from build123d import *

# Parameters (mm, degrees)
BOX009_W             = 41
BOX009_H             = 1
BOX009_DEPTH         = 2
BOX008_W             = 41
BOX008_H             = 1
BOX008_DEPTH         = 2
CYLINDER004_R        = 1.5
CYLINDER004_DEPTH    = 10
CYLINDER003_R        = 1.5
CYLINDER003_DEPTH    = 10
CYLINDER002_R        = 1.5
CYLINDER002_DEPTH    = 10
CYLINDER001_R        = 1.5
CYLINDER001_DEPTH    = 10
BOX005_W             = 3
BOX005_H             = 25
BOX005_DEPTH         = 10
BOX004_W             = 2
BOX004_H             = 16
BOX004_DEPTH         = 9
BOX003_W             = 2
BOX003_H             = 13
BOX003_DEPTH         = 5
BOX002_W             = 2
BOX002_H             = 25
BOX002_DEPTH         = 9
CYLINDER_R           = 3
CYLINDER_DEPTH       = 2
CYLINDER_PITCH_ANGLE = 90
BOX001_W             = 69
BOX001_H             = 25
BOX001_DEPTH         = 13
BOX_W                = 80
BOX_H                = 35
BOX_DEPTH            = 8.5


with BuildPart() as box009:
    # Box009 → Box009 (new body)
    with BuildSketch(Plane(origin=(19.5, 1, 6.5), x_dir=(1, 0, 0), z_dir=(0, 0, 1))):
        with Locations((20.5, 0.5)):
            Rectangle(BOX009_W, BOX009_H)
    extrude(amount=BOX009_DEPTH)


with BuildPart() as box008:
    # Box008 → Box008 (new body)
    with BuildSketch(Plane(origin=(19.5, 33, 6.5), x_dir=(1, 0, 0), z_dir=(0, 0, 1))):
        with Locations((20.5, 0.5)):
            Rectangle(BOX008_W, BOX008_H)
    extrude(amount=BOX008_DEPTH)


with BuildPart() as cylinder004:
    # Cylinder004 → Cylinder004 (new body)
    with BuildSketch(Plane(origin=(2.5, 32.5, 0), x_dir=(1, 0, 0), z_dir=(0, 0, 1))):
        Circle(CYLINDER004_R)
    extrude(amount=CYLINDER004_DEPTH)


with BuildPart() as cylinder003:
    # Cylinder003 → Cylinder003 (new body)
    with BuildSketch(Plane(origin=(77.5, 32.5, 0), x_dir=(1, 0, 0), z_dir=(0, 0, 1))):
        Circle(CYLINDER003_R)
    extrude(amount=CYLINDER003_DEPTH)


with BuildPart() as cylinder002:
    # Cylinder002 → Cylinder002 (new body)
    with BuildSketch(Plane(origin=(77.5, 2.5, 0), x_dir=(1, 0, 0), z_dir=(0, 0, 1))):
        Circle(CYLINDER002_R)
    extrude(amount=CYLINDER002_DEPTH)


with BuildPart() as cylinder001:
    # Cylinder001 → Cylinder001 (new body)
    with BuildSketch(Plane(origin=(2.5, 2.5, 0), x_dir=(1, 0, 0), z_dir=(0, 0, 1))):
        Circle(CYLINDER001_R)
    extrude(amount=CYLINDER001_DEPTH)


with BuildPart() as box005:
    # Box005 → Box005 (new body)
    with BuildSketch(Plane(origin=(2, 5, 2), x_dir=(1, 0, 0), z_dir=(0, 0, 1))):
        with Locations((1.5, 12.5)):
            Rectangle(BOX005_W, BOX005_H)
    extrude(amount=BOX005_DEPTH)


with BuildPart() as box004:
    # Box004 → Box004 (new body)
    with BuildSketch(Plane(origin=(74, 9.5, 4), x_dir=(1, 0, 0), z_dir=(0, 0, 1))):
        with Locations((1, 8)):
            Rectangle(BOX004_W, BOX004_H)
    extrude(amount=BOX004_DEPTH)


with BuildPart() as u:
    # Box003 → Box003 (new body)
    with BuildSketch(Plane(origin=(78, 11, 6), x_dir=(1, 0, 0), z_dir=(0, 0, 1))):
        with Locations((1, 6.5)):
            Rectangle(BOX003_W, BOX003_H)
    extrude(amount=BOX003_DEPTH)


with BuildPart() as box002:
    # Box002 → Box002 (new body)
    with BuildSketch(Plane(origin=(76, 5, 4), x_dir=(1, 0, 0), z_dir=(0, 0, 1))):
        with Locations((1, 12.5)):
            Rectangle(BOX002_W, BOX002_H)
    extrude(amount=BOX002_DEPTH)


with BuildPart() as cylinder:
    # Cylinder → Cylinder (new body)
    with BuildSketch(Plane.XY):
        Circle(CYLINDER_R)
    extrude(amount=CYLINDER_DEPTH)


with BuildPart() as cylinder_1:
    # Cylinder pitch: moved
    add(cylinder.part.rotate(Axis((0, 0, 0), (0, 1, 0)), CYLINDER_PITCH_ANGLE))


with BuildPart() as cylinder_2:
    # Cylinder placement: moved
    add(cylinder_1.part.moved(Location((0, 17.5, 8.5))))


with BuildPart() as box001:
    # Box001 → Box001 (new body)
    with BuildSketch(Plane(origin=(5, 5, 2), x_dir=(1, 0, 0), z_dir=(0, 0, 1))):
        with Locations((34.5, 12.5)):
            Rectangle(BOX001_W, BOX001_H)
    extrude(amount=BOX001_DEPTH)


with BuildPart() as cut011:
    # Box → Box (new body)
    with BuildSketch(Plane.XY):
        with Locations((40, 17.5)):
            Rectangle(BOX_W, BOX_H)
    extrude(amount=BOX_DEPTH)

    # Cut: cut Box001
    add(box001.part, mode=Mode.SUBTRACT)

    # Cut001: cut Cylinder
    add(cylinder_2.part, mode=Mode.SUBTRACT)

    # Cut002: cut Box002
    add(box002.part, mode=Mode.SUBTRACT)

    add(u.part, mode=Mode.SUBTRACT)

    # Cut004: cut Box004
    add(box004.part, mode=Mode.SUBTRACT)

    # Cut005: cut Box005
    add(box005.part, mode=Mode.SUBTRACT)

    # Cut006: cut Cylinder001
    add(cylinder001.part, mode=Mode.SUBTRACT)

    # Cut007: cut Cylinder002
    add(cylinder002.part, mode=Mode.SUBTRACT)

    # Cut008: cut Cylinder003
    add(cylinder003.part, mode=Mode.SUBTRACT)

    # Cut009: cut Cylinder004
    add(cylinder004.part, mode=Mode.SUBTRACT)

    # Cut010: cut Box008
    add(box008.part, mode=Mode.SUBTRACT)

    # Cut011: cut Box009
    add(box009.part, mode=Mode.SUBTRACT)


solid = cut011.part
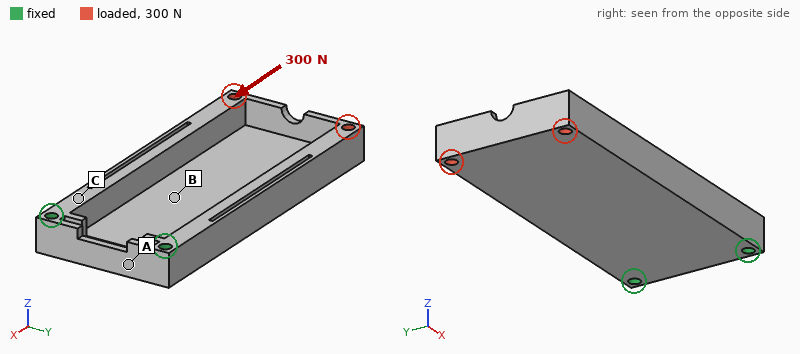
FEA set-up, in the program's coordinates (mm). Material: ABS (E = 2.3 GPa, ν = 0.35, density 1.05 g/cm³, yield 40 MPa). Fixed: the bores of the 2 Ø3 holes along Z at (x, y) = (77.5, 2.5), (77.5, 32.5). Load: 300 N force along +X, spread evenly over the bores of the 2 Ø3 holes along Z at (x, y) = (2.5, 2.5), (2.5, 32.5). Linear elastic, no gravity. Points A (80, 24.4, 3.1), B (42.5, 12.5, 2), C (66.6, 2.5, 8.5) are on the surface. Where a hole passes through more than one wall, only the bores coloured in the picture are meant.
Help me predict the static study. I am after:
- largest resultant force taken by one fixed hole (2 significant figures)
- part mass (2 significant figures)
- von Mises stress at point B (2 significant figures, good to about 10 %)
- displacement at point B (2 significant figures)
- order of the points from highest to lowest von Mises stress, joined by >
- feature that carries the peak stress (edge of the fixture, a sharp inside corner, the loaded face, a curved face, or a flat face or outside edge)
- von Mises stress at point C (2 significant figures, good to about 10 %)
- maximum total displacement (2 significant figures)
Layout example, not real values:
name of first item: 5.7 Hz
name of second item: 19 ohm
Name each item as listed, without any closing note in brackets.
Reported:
largest resultant force taken by one fixed hole: 150 N
part mass: 12 g
von Mises stress at point B: 1.8 MPa
displacement at point B: 0.086 mm
order of the points from highest to lowest von Mises stress, joined by >: C > B > A
feature that carries the peak stress: the loaded face
von Mises stress at point C: 4.3 MPa
maximum total displacement: 0.55 mm
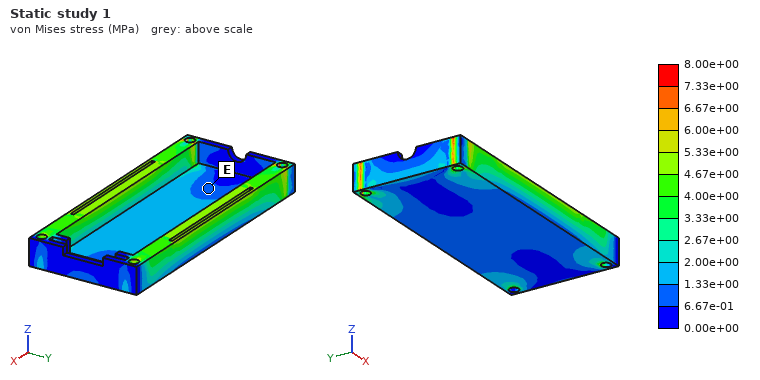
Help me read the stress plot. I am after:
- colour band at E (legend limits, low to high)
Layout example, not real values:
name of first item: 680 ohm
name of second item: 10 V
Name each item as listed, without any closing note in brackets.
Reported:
colour band at E: 6.67e-01 to 1.33e+00 MPa
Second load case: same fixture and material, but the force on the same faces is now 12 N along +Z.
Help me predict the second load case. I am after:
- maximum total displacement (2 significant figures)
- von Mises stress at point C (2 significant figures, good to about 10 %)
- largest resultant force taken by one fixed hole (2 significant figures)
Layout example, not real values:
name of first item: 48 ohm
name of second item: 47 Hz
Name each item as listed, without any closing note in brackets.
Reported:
maximum total displacement: 1.0 mm
von Mises stress at point C: 5.2 MPa
largest resultant force taken by one fixed hole: 16 N
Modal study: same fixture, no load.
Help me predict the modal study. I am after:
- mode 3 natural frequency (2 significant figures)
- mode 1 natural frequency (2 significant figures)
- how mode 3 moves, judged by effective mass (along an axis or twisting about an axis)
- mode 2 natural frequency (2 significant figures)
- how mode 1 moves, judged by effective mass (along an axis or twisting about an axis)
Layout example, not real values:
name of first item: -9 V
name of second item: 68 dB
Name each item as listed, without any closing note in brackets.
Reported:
mode 3 natural frequency: 1400 Hz
mode 1 natural frequency: 310 Hz
how mode 3 moves, judged by effective mass: along Y
mode 2 natural frequency: 590 Hz
how mode 1 moves, judged by effective mass: along Z
